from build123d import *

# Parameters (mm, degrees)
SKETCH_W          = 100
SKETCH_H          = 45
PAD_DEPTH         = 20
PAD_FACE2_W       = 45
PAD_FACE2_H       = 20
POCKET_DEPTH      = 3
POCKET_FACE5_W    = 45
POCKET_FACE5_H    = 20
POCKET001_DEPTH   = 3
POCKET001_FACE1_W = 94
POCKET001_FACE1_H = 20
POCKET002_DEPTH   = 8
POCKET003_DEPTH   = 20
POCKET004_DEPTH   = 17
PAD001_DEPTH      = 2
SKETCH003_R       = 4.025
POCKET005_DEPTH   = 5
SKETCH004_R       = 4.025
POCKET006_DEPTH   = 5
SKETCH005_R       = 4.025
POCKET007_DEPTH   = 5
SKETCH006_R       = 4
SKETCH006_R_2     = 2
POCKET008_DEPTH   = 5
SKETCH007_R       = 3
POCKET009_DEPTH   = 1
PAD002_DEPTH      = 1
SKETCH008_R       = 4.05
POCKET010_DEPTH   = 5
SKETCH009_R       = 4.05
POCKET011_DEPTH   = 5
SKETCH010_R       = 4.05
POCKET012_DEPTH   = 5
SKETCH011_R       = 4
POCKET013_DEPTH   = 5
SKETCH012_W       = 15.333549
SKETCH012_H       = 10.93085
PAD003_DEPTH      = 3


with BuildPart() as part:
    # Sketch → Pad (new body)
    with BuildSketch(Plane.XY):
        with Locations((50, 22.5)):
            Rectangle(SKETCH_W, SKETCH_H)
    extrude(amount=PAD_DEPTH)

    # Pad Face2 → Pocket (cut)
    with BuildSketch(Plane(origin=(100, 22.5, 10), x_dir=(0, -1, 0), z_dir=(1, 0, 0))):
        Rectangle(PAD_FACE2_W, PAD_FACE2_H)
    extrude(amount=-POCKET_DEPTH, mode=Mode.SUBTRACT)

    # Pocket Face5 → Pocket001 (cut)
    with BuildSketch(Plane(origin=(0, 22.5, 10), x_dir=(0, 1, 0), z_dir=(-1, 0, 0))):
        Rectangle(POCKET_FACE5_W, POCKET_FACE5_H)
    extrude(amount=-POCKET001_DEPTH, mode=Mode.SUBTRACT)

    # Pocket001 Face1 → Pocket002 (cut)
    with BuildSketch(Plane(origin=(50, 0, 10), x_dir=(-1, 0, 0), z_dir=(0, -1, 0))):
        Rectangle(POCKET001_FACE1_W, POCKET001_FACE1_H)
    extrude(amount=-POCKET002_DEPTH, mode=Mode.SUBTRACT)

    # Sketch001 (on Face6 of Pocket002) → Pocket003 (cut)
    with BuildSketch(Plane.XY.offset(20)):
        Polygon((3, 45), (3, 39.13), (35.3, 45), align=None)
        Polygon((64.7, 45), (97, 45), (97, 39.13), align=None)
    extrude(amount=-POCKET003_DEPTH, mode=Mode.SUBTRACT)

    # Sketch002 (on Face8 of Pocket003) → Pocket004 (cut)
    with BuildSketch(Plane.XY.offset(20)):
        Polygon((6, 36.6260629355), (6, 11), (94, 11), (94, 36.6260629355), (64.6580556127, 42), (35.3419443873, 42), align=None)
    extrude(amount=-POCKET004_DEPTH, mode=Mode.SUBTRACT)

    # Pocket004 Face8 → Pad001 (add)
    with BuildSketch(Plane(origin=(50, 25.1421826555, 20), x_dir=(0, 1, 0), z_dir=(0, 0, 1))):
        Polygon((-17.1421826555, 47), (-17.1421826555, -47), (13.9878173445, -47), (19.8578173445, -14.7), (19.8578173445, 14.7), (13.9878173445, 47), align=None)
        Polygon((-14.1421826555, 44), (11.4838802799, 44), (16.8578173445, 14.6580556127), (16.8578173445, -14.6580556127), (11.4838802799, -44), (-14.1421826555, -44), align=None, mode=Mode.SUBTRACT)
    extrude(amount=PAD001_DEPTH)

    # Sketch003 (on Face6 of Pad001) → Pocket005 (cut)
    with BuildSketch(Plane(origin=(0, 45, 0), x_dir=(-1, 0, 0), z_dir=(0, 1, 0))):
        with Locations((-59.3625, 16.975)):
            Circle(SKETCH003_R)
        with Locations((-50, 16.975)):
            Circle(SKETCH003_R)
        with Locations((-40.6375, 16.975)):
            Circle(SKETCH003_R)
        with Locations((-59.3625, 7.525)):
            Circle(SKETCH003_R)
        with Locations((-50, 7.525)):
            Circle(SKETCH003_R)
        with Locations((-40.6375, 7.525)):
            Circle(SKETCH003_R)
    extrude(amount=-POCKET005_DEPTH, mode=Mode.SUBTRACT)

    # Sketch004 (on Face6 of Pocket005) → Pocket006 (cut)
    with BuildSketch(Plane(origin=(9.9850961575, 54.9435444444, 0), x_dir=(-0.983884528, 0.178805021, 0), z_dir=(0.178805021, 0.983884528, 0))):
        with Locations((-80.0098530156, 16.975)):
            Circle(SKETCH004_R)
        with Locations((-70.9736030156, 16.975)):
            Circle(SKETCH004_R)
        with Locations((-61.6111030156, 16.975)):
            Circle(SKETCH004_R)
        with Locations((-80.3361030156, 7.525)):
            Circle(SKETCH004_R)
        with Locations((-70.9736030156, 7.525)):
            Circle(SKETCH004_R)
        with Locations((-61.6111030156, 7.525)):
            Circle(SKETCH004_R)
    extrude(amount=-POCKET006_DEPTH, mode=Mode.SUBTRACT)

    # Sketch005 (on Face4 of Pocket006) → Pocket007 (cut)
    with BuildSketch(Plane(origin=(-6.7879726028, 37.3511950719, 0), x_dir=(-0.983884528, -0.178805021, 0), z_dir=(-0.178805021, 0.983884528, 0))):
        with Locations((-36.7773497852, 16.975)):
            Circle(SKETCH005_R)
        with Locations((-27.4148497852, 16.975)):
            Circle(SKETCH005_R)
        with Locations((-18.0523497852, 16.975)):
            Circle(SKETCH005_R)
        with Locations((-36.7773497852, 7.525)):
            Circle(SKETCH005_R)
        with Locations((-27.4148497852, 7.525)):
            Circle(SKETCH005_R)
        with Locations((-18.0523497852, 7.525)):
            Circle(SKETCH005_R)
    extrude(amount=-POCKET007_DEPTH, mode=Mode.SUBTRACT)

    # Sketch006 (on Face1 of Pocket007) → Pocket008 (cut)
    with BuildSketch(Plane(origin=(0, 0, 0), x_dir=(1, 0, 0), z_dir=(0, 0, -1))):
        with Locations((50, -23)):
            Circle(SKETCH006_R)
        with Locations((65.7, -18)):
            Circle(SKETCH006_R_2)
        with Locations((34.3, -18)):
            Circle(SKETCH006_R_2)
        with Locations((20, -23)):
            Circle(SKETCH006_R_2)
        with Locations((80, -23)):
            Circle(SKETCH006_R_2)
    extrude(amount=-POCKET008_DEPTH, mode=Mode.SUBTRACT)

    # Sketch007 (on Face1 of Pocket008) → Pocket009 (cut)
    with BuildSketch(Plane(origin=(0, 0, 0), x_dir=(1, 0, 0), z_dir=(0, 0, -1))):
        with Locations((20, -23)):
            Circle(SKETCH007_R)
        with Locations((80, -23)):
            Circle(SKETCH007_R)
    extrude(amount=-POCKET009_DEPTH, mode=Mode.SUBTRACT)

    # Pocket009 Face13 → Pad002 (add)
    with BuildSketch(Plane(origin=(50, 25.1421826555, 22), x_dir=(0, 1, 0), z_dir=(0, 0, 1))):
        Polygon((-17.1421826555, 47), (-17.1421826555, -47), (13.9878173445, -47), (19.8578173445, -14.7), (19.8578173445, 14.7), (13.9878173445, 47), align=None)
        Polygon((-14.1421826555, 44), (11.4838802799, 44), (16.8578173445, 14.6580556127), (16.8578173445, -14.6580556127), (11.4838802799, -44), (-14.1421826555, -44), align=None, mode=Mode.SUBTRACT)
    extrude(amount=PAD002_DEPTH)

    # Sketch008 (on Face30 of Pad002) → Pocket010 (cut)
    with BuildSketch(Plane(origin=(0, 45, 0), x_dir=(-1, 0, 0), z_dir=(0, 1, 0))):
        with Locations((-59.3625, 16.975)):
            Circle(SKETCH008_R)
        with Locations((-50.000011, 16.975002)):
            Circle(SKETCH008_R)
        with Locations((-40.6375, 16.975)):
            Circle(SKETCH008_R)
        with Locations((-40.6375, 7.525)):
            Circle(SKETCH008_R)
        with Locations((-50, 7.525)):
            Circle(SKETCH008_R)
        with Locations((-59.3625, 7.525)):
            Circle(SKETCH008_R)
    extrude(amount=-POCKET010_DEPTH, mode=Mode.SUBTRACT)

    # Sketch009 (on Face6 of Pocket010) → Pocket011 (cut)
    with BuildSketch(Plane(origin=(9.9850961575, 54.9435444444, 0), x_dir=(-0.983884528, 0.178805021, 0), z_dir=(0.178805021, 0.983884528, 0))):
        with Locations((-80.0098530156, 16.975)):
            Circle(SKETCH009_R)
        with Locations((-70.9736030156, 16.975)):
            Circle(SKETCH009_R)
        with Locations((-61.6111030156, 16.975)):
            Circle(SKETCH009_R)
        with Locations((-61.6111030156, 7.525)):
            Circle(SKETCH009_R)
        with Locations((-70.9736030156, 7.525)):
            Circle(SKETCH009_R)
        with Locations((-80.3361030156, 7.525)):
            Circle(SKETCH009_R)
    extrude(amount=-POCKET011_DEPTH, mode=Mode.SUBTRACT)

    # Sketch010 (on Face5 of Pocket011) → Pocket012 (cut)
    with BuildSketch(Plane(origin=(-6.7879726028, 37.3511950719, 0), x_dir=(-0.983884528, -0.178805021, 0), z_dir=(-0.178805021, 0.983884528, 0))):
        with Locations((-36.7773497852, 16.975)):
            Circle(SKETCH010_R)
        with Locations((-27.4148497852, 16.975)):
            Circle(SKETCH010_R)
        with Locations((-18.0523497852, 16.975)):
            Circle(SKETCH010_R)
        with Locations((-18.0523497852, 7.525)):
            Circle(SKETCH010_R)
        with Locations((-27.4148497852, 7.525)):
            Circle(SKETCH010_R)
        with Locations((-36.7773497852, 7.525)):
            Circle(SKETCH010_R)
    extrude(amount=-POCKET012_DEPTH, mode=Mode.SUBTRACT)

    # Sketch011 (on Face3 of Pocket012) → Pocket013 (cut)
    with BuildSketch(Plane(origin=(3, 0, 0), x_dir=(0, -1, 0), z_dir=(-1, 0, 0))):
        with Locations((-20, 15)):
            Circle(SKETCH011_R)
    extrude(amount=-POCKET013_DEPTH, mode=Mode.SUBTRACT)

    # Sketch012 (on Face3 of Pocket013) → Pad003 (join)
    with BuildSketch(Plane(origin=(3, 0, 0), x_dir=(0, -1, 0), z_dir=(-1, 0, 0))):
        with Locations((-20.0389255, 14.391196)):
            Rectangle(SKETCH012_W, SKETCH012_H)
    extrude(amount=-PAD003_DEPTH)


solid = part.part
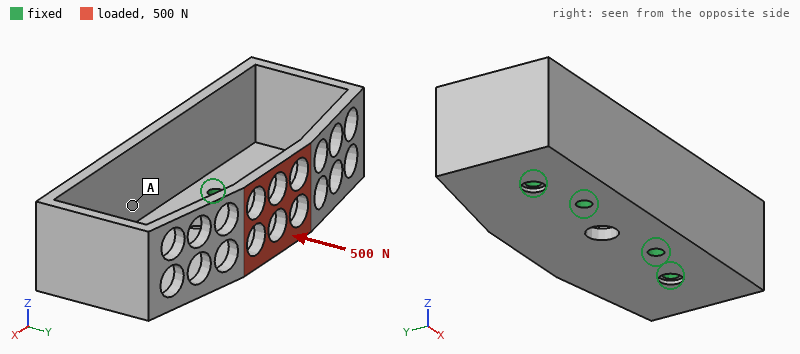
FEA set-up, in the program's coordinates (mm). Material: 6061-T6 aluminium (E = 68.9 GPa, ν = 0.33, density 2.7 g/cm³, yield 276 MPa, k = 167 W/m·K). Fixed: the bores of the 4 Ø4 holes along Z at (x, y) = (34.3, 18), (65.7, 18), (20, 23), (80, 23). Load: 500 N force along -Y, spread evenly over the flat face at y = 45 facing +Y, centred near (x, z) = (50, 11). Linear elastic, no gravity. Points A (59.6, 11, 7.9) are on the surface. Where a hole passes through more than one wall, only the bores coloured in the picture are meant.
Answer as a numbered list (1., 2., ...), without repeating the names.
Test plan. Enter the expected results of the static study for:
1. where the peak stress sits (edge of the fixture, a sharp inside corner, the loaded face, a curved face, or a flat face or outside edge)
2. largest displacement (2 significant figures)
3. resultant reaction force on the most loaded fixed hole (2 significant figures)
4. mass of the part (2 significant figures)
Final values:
1. a curved face
2. 0.32 mm
3. 190 N
4. 57 g
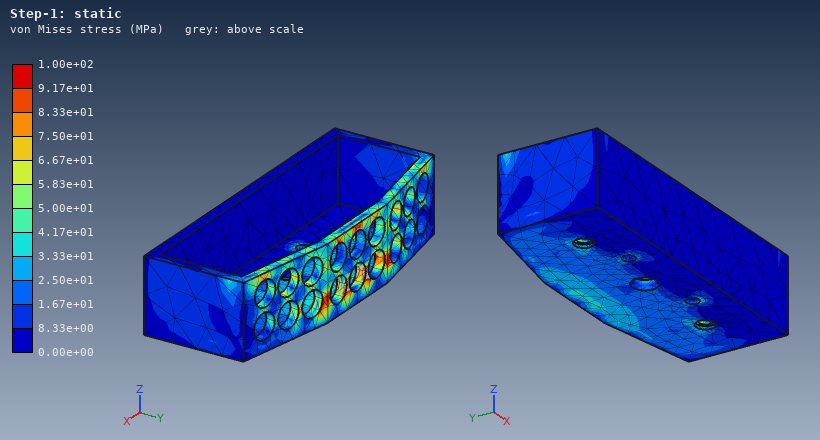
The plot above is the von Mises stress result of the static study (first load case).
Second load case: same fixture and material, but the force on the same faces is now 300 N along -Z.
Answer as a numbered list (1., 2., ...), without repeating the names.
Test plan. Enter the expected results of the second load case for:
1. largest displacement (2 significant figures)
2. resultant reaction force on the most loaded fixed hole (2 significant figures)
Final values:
1. 0.17 mm
2. 230 N
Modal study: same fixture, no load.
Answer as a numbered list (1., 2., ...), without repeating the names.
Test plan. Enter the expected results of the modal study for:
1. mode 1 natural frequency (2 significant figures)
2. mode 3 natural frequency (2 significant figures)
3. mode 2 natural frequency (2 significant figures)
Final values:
1. 2500 Hz
2. 3700 Hz
3. 2800 Hz
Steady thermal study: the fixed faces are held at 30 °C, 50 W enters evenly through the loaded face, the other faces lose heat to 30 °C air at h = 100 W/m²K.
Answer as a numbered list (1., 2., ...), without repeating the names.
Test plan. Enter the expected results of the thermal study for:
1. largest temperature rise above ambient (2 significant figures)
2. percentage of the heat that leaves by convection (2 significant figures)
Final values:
1. 74 K
2. 34 %
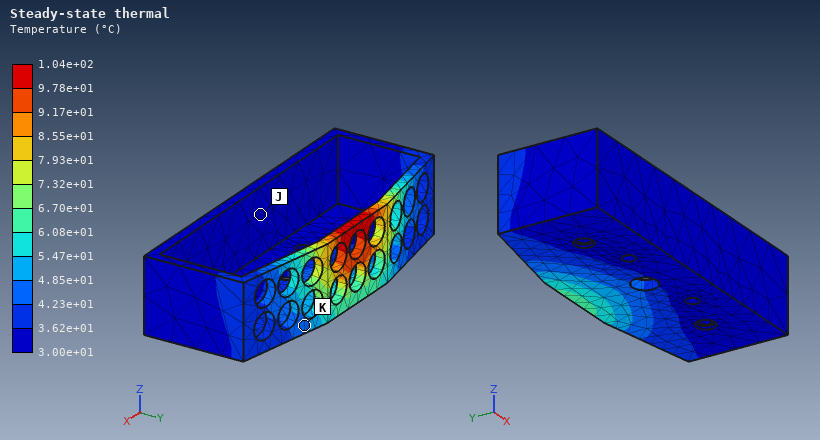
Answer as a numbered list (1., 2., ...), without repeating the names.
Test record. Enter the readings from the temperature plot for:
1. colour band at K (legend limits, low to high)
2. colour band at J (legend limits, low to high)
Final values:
1. 4.23e+01 to 4.85e+01 °C
2. 3.00e+01 to 3.62e+01 °C
